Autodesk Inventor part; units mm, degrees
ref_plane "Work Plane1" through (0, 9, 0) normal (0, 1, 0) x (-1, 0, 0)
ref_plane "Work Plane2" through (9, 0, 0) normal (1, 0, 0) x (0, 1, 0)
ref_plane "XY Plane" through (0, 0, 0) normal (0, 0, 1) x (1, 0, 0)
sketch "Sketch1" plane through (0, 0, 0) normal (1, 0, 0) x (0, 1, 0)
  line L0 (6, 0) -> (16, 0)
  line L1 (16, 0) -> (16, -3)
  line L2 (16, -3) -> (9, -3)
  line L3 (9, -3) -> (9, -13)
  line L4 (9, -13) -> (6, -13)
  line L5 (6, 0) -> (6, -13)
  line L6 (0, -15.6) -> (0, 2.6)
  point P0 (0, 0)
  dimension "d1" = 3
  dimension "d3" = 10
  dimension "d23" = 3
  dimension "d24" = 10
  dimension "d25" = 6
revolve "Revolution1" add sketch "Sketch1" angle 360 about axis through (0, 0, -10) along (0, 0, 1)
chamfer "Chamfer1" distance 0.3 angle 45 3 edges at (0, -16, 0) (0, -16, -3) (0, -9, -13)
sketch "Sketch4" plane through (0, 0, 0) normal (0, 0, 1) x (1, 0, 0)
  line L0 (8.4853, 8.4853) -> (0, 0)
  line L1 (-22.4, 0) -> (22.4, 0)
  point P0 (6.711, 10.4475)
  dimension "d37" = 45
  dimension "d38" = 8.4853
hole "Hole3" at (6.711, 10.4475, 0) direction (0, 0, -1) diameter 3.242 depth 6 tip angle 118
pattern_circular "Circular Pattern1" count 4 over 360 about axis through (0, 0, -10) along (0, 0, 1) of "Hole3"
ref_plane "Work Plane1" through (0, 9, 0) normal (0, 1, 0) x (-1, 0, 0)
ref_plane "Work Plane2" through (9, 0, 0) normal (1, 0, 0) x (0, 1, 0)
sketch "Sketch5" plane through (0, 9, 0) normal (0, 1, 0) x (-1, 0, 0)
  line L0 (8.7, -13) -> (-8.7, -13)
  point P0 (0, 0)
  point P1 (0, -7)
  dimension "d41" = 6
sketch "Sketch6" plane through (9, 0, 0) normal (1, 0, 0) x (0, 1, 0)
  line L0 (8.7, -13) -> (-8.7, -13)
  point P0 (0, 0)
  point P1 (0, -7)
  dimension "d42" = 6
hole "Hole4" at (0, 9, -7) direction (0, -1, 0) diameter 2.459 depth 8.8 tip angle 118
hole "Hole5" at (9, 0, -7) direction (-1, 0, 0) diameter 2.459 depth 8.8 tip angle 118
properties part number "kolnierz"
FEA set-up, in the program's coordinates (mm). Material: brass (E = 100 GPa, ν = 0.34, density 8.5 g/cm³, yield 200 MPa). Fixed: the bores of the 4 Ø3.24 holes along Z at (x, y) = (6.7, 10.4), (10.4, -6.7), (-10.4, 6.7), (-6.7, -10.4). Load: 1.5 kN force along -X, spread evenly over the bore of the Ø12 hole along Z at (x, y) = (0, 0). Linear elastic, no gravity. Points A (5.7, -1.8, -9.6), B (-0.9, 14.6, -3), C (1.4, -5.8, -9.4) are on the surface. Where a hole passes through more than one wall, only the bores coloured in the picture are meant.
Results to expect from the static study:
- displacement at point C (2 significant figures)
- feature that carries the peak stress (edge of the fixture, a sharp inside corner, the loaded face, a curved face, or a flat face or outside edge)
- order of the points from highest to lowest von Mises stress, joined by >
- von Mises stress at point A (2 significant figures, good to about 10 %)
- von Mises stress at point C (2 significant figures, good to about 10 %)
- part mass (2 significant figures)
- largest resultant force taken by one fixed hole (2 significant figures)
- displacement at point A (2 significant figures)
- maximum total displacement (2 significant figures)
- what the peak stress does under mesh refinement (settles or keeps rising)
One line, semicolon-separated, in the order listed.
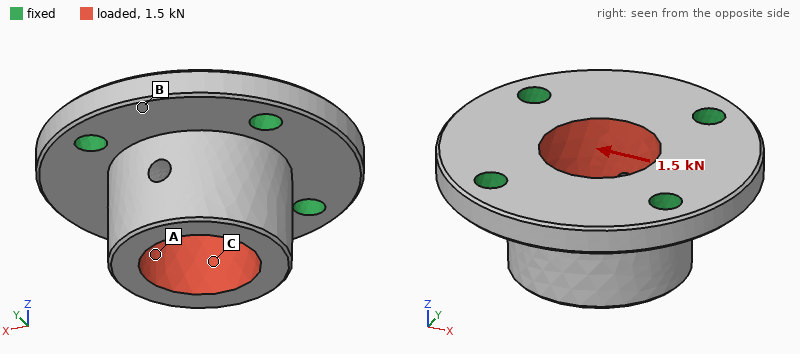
4.1 µm; edge of the fixture; C > A > B; 8.8 MPa; 18 MPa; 28 g; 490 N; 4.7 µm; 6.6 µm; keeps rising
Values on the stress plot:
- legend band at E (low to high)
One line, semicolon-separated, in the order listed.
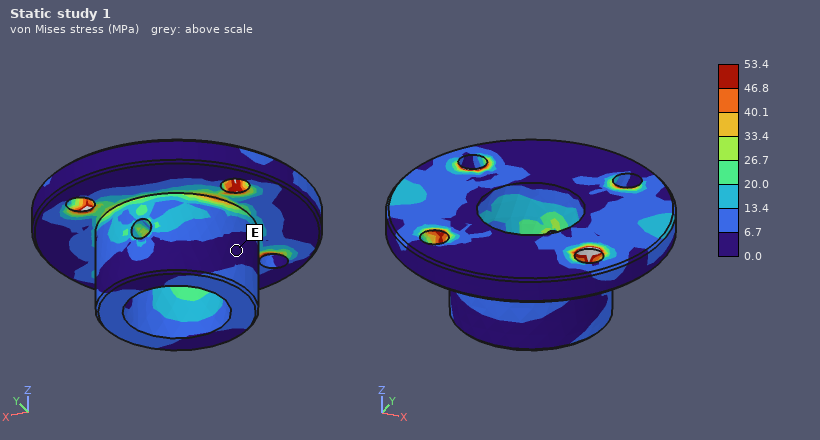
0.0 to 6.7 MPa
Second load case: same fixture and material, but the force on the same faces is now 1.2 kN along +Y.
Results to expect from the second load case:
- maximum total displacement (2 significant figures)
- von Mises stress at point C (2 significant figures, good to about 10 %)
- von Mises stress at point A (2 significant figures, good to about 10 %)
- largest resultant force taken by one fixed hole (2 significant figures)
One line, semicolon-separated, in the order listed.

5.3 µm; 4.4 MPa; 12 MPa; 400 N
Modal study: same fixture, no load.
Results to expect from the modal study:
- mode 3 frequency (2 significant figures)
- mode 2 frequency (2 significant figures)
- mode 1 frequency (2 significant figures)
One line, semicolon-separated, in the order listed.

25 kHz; 21 kHz; 21 kHz
